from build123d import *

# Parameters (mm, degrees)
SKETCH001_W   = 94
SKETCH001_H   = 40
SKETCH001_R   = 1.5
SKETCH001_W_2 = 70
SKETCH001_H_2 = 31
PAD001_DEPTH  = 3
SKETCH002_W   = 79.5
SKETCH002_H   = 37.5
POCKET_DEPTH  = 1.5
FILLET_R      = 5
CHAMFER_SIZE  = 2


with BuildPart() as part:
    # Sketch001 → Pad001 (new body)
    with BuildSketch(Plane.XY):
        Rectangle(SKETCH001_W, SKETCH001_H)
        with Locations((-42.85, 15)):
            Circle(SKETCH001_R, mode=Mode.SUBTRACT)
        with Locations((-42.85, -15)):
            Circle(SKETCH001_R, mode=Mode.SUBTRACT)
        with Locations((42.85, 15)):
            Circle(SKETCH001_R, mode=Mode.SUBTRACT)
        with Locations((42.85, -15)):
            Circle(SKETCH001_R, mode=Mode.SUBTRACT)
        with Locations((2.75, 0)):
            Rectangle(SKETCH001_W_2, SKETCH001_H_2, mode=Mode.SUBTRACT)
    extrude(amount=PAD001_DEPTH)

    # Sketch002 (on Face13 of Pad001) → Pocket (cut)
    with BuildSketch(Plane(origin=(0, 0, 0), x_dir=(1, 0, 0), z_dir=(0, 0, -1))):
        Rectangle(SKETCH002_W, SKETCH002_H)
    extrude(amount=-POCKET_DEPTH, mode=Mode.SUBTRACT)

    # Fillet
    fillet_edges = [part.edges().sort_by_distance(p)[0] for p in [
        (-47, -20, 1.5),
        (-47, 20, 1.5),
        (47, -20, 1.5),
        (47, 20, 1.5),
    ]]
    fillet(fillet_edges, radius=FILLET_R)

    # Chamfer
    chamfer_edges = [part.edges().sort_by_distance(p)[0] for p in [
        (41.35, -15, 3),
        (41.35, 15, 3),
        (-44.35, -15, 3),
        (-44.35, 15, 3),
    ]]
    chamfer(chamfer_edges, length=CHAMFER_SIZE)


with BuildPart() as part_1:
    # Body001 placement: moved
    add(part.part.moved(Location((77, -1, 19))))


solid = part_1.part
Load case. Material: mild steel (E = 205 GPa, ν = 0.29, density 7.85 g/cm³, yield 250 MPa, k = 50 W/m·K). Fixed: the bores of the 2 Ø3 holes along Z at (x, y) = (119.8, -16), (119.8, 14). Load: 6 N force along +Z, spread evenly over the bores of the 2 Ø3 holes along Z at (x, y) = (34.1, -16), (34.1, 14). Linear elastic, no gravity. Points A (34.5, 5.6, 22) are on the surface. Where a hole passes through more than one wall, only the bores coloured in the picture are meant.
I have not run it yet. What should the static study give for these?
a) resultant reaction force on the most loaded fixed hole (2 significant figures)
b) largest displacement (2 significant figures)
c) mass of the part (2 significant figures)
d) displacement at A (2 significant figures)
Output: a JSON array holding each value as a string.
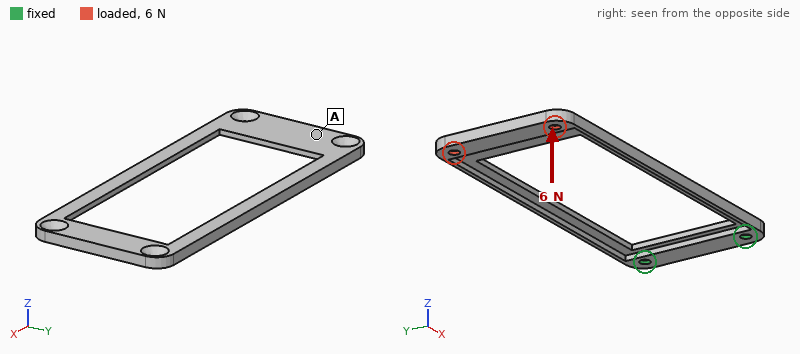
["11 N", "0.68 mm", "26 g", "0.63 mm"]
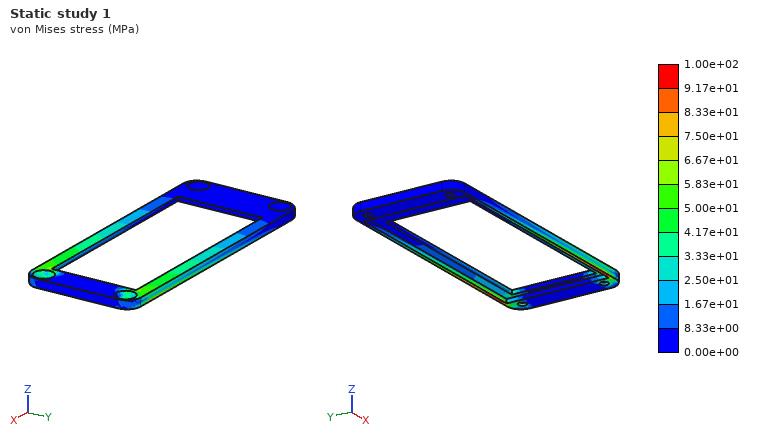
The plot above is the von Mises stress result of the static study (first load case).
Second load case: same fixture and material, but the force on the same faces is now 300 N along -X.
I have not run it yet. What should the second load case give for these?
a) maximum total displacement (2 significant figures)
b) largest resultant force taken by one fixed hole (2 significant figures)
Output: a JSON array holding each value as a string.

["0.84 mm", "150 N"]
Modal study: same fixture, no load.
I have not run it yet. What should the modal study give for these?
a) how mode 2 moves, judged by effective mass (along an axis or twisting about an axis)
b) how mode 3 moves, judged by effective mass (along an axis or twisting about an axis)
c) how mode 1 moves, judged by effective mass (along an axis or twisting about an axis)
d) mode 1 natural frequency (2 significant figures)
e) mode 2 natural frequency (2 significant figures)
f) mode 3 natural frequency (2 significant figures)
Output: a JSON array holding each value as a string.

["along Y", "along Y", "along Z", "150 Hz", "450 Hz", "630 Hz"]
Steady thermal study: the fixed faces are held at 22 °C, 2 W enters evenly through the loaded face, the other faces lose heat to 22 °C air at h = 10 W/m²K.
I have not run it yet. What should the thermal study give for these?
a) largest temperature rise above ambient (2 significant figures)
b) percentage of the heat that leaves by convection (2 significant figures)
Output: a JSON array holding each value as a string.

["69 K", "75 %"]
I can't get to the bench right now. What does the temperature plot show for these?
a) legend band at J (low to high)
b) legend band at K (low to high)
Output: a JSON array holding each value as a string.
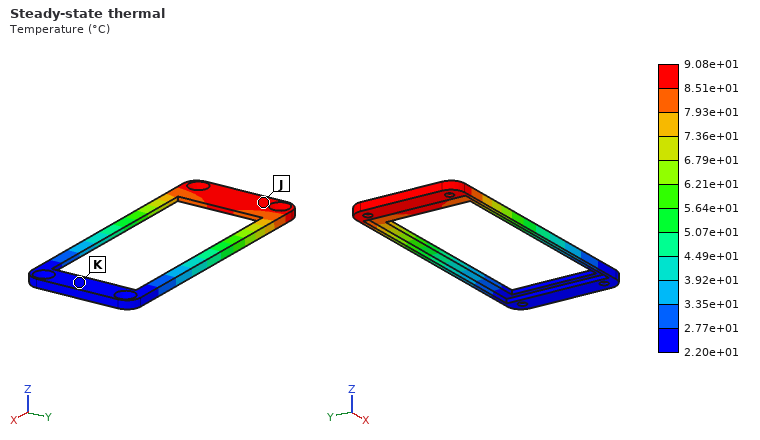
["8.51e+01 to 9.08e+01 °C", "2.20e+01 to 2.77e+01 °C"]
